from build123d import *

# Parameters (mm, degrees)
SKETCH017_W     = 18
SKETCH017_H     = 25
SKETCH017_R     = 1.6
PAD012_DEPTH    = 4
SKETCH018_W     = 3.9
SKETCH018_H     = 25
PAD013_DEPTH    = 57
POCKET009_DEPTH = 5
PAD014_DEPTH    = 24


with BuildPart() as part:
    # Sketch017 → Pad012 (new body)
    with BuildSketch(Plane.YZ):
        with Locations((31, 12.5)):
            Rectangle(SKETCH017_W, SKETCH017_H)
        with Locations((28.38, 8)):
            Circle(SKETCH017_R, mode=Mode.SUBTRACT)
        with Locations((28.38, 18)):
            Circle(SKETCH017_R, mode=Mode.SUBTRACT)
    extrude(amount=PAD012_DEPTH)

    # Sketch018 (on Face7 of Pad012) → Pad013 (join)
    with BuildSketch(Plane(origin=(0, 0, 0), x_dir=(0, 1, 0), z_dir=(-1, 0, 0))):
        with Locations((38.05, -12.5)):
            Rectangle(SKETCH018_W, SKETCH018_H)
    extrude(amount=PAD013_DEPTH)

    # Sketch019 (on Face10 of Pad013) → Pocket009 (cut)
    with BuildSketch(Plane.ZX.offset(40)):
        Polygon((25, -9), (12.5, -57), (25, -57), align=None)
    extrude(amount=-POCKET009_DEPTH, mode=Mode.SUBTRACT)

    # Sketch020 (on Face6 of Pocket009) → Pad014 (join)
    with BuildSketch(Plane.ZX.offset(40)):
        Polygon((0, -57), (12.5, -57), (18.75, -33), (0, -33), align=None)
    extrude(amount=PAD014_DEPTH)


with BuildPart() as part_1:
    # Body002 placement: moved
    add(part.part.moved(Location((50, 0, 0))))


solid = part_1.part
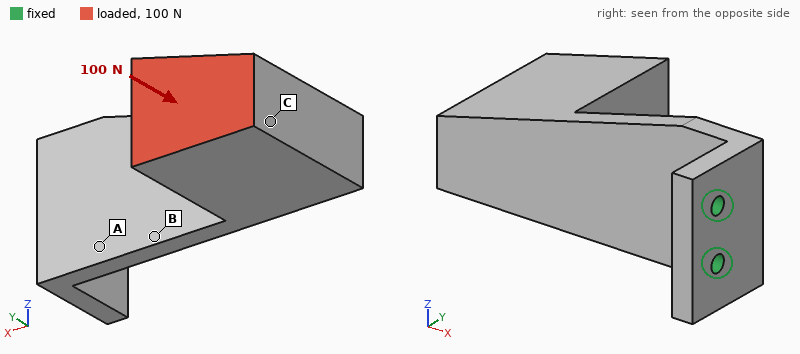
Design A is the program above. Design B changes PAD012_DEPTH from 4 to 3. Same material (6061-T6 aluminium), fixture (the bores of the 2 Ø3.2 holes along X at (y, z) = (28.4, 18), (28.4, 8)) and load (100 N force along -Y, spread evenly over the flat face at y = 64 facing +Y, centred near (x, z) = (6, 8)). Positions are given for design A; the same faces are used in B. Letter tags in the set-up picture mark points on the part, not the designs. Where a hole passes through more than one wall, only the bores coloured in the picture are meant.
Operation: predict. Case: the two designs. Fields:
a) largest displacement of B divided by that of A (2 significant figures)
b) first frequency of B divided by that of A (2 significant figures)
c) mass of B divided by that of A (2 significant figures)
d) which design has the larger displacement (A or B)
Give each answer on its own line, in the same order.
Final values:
1.4
0.85
0.97
B
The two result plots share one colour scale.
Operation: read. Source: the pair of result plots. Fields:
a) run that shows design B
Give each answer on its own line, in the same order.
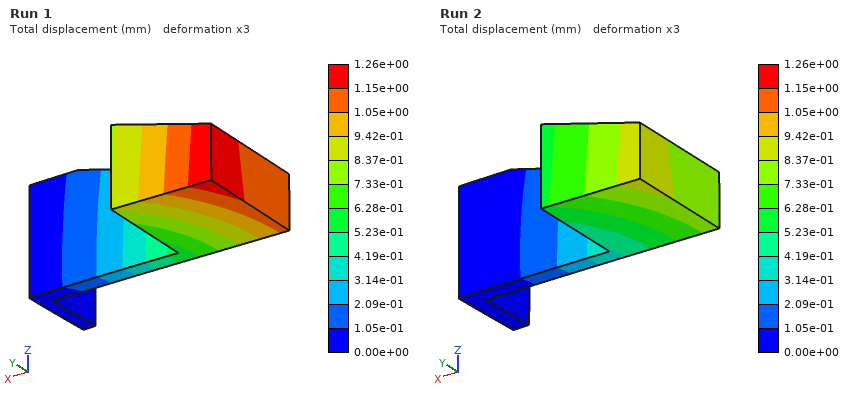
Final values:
Run 1
